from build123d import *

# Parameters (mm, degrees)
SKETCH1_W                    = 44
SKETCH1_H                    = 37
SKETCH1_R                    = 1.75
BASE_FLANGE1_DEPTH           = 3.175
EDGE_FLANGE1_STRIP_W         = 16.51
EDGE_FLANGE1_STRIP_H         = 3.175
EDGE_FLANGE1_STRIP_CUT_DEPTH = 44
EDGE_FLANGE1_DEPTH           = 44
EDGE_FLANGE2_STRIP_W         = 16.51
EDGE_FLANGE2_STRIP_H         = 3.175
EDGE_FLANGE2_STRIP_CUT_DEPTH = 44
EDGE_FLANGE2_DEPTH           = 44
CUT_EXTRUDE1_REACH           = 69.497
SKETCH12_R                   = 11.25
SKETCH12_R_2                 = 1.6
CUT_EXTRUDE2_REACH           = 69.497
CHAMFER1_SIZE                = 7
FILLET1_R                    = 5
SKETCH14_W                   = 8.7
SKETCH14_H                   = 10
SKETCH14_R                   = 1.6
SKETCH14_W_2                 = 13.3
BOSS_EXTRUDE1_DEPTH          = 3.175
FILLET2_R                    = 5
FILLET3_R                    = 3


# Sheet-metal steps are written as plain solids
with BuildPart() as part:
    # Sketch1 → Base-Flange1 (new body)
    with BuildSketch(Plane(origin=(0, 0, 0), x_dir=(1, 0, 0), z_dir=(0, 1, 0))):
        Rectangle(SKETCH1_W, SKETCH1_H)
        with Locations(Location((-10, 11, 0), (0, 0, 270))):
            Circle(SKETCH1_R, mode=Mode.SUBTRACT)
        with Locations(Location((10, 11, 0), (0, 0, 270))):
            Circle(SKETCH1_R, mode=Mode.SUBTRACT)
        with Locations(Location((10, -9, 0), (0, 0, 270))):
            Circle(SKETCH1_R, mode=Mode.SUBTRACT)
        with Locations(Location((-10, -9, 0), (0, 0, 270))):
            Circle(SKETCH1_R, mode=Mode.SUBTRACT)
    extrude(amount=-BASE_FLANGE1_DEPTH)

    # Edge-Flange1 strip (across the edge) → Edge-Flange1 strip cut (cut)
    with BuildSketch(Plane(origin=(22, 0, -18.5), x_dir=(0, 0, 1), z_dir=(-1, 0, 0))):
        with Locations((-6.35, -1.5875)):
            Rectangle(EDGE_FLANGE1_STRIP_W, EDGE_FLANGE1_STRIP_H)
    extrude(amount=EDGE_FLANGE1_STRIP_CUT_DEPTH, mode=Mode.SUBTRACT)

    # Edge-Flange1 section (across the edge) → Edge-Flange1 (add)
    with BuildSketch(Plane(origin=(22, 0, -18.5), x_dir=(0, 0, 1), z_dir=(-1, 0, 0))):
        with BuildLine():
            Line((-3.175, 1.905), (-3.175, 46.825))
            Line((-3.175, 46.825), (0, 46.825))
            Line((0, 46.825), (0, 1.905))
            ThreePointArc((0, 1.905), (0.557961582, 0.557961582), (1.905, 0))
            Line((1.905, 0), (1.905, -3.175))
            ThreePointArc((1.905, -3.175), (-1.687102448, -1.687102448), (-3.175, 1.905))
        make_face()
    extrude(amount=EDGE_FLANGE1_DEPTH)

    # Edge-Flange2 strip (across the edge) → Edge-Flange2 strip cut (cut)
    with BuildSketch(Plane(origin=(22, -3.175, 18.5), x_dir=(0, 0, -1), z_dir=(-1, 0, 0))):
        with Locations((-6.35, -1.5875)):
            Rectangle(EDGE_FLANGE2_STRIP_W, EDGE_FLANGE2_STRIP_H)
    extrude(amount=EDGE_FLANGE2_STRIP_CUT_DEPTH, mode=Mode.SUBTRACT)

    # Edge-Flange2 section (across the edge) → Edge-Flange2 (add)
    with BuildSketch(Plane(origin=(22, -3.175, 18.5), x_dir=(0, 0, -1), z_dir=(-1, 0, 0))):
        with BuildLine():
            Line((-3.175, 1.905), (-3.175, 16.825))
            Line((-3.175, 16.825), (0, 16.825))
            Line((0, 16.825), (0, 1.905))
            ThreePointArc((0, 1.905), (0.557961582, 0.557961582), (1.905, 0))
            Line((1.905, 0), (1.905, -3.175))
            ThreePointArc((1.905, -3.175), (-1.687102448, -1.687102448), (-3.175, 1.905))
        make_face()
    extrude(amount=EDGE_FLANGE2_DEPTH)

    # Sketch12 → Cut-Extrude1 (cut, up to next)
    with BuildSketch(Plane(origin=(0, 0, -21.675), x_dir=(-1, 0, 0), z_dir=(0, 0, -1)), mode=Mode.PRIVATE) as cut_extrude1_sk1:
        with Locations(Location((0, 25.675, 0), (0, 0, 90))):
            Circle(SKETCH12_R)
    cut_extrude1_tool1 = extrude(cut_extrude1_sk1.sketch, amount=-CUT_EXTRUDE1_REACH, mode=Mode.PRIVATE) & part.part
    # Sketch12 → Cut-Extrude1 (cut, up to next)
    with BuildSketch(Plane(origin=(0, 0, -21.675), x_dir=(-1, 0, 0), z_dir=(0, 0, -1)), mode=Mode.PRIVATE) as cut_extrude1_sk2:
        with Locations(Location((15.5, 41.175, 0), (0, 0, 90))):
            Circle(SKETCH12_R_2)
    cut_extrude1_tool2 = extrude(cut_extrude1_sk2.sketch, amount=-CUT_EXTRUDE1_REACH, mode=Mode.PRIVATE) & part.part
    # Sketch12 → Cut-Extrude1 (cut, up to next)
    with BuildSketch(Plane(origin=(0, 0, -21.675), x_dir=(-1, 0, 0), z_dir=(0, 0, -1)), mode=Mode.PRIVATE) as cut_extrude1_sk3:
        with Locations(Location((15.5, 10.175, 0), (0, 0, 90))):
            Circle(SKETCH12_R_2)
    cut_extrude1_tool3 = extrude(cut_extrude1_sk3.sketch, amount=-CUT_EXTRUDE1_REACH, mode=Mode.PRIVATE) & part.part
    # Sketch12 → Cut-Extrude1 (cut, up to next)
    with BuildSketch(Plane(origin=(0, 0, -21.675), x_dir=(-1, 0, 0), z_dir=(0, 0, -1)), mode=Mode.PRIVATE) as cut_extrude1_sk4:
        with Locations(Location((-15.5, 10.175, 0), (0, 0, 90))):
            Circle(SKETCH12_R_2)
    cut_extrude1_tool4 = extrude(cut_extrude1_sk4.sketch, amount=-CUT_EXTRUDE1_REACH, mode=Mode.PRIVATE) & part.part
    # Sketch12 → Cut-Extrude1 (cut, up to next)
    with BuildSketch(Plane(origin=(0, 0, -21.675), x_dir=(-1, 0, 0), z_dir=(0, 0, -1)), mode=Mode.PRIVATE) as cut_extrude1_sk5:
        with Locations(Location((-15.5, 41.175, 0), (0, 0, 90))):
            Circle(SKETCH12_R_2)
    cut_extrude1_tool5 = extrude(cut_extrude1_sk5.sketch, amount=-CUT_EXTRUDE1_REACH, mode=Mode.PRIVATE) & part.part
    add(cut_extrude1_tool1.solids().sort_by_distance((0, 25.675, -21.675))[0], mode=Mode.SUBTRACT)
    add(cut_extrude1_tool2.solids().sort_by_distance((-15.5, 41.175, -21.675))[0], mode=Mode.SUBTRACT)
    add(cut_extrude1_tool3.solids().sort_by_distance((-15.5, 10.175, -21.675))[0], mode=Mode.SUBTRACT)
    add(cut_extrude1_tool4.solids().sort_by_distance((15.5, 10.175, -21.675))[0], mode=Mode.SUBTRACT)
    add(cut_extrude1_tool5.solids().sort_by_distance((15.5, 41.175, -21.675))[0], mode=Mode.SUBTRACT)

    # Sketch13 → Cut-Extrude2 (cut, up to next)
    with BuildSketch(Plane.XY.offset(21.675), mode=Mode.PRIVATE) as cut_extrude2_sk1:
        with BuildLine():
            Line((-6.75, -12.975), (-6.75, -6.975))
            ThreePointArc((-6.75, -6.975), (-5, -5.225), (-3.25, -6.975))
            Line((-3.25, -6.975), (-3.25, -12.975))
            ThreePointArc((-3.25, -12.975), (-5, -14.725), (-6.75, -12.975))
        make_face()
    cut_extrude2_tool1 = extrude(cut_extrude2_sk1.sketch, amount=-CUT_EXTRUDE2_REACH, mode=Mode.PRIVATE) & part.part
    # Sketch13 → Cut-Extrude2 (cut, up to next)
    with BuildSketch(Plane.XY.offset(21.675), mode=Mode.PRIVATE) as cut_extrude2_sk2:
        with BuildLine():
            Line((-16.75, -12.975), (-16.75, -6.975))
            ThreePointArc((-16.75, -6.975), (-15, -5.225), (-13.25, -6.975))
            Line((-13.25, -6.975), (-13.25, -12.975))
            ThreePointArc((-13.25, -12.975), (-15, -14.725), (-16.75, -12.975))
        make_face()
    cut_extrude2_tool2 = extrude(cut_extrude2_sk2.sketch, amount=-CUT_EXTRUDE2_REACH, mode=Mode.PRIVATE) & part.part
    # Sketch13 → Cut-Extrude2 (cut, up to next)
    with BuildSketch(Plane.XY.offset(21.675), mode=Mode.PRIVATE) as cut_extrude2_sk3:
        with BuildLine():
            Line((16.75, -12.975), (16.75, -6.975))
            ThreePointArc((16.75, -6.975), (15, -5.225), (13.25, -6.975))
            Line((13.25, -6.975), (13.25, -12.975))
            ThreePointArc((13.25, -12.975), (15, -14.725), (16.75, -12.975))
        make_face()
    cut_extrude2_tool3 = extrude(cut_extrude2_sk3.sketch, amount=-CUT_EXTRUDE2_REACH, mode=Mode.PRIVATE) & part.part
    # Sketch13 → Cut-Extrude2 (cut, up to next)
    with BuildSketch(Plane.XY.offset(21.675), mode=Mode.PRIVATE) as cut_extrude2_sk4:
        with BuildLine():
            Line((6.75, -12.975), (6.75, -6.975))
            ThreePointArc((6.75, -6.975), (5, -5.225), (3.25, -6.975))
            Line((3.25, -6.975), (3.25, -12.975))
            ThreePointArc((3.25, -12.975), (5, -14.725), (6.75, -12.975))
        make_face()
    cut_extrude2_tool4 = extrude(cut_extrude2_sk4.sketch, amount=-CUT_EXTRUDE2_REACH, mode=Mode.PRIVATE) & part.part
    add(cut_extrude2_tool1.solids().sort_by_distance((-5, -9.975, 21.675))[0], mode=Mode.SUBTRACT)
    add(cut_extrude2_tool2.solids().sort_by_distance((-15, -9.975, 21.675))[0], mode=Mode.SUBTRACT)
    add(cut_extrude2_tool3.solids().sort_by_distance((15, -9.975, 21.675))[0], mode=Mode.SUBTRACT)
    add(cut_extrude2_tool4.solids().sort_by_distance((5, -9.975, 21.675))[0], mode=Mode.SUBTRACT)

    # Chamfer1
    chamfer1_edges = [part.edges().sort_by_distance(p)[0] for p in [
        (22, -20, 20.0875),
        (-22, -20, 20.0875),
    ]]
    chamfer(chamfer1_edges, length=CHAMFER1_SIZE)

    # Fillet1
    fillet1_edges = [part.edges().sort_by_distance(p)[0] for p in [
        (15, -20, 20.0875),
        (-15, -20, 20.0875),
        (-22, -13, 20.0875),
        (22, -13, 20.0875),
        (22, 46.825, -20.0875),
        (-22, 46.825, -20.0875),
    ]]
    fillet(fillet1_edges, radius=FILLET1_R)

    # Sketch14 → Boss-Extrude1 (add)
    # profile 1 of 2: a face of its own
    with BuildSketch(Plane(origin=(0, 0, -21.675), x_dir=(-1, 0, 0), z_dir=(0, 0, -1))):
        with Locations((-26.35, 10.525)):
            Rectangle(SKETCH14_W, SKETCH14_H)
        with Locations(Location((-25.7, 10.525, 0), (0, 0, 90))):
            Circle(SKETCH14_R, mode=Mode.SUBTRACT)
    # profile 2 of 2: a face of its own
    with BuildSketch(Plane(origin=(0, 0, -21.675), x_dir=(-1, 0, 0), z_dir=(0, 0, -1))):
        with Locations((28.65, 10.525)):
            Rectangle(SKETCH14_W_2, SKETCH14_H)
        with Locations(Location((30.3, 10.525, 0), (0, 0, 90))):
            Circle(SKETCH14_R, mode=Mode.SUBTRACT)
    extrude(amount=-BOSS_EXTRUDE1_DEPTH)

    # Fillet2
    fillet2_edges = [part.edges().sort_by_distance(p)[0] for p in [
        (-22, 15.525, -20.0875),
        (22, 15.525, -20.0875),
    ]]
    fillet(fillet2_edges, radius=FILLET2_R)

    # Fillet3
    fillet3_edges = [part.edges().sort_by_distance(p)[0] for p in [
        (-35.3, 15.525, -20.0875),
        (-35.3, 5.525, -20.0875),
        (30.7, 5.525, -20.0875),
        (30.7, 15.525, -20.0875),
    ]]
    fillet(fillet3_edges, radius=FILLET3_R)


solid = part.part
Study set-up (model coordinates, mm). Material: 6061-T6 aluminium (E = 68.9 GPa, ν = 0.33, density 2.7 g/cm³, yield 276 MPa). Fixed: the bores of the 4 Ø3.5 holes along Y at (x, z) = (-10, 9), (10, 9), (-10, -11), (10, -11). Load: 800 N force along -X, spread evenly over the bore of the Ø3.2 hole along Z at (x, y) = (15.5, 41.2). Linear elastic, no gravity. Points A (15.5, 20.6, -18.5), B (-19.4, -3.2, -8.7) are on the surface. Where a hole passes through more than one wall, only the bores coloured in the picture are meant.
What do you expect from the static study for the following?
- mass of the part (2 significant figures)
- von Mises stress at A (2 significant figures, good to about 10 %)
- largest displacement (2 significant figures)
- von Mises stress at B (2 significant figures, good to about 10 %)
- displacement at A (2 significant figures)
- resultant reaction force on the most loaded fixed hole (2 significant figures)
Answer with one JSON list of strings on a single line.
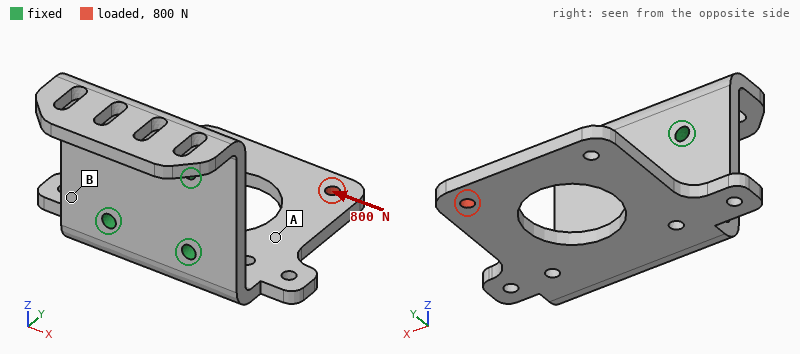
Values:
["35 g", "42 MPa", "0.39 mm", "89 MPa", "0.20 mm", "1.6 kN"]
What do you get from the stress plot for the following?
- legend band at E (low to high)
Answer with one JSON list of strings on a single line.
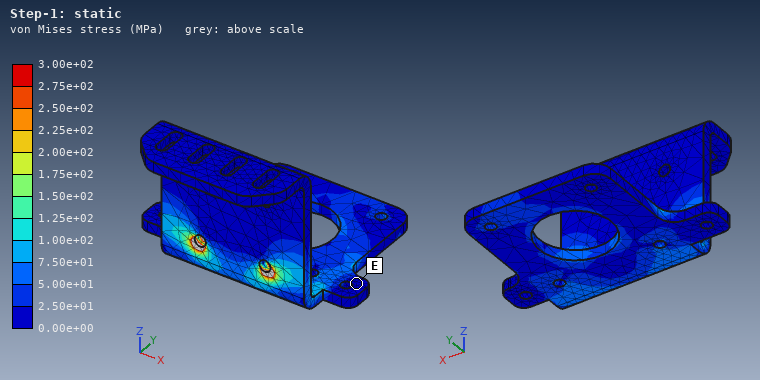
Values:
["0.00e+00 to 2.50e+01 MPa"]
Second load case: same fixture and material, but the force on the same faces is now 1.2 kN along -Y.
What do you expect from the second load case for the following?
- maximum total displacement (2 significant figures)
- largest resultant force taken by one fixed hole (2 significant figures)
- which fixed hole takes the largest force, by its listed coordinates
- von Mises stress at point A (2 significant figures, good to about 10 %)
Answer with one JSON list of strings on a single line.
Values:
["0.44 mm", "1.5 kN", "(10, -11)", "37 MPa"]
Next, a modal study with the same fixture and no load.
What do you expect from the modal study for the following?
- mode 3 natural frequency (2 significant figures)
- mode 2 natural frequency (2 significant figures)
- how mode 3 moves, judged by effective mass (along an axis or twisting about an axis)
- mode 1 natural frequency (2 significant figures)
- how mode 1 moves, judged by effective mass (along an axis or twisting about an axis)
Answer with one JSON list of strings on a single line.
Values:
["3300 Hz", "2200 Hz", "along X", "920 Hz", "along Z"]
